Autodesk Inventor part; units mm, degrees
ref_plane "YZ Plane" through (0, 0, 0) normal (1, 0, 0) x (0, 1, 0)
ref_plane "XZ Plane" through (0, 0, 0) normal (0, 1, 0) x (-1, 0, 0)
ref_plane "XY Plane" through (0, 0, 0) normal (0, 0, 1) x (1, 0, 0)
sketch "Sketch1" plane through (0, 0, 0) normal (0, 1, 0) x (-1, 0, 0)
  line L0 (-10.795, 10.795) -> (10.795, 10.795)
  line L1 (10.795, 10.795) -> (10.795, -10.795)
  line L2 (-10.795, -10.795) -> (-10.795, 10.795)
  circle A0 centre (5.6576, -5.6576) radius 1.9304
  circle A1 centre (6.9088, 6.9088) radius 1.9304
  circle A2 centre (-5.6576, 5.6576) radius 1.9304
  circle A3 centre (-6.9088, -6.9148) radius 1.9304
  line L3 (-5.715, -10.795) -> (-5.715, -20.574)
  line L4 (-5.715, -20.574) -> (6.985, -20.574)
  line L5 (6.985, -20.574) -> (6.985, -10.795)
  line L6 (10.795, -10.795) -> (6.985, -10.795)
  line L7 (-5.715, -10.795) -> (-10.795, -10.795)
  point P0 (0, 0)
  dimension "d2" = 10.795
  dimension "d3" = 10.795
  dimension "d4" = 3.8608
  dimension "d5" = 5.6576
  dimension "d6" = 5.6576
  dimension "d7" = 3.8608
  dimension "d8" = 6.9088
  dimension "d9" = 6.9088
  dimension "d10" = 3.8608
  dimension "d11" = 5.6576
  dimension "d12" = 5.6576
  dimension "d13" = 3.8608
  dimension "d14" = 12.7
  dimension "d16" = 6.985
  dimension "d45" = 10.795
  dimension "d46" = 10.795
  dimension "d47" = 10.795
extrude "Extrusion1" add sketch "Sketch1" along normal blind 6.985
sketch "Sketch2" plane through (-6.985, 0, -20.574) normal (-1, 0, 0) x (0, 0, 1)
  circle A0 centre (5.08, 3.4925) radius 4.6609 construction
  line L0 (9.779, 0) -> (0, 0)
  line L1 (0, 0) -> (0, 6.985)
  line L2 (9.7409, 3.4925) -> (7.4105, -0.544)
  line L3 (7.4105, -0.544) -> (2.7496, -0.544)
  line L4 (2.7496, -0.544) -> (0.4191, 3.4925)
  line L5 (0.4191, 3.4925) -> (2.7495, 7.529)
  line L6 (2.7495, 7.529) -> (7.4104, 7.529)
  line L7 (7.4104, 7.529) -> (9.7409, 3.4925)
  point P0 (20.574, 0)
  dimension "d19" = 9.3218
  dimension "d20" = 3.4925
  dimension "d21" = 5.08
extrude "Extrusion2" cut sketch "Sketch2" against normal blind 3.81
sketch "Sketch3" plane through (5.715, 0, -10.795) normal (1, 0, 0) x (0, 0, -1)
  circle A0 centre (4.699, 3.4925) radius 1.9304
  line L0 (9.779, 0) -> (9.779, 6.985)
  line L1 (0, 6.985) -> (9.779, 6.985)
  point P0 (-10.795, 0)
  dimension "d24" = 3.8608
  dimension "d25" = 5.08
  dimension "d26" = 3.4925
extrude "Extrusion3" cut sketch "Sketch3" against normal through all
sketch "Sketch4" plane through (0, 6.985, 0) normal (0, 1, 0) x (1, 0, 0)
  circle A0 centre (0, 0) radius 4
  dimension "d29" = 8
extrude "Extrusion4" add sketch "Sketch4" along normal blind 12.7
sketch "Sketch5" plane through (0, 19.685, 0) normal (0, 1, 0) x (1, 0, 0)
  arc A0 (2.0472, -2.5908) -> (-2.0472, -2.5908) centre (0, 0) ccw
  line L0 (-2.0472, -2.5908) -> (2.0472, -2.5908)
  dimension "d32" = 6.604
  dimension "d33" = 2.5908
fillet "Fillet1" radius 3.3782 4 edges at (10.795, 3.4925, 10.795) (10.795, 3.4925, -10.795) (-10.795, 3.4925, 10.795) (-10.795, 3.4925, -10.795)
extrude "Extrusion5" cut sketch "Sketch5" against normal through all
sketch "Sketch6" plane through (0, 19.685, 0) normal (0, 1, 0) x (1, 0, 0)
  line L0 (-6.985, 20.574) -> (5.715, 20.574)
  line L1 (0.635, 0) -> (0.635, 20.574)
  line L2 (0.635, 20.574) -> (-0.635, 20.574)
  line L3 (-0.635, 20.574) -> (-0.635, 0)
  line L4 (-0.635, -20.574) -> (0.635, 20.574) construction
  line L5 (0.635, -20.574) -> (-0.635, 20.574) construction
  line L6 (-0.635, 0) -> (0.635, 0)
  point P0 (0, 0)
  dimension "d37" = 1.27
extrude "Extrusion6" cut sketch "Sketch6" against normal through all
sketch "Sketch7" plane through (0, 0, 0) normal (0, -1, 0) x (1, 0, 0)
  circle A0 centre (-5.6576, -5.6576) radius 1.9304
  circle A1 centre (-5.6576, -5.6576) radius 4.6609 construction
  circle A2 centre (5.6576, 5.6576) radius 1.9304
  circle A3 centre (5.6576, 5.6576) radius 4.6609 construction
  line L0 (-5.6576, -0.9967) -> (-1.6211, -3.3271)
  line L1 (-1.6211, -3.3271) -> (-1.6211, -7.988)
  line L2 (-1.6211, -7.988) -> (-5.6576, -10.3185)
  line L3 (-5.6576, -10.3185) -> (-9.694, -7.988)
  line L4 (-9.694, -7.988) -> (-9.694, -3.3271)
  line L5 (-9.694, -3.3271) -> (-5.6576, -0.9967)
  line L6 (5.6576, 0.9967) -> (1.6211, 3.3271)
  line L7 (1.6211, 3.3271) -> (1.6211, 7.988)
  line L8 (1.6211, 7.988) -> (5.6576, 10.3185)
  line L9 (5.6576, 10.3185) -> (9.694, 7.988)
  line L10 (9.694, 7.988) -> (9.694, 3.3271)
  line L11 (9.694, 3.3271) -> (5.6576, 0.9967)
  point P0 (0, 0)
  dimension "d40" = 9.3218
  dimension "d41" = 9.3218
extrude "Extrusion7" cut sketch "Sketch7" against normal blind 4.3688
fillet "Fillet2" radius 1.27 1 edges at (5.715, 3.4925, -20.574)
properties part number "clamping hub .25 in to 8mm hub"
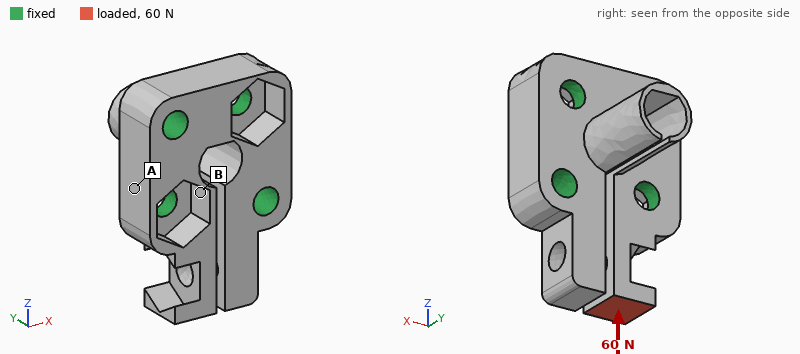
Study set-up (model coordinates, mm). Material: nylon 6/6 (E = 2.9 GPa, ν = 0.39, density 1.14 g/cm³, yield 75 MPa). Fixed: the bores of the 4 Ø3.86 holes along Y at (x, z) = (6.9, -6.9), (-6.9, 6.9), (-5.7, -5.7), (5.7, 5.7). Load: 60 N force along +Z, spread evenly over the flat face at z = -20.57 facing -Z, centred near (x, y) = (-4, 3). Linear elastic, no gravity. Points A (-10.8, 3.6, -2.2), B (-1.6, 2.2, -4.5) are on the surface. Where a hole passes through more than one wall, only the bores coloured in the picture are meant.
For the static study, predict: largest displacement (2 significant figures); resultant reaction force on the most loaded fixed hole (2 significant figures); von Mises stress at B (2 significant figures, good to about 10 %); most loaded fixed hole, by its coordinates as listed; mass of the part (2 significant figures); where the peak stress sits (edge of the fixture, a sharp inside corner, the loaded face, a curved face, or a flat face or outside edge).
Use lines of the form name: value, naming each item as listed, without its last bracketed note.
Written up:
largest displacement: 0.51 mm
resultant reaction force on the most loaded fixed hole: 53 N
von Mises stress at B: 4.9 MPa
most loaded fixed hole, by its coordinates as listed: (-5.7, -5.7)
mass of the part: 3.3 g
where the peak stress sits: a curved face
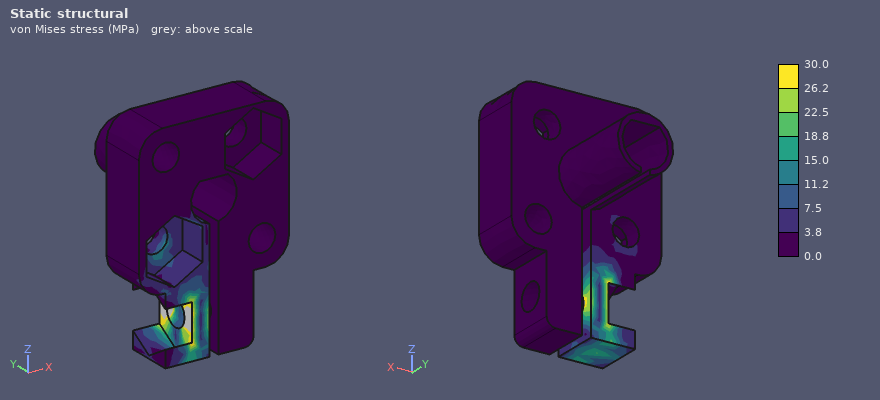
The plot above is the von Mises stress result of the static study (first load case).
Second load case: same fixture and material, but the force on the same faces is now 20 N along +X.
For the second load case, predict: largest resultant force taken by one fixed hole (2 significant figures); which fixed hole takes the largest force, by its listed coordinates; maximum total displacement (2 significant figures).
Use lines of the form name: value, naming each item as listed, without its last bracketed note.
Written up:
largest resultant force taken by one fixed hole: 30 N
which fixed hole takes the largest force, by its listed coordinates: (-5.7, -5.7)
maximum total displacement: 0.51 mm
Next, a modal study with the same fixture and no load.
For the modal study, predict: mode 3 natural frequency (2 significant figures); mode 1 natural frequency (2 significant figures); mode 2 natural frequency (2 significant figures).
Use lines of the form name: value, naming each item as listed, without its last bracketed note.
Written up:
mode 3 natural frequency: 4400 Hz
mode 1 natural frequency: 3700 Hz
mode 2 natural frequency: 4300 Hz
